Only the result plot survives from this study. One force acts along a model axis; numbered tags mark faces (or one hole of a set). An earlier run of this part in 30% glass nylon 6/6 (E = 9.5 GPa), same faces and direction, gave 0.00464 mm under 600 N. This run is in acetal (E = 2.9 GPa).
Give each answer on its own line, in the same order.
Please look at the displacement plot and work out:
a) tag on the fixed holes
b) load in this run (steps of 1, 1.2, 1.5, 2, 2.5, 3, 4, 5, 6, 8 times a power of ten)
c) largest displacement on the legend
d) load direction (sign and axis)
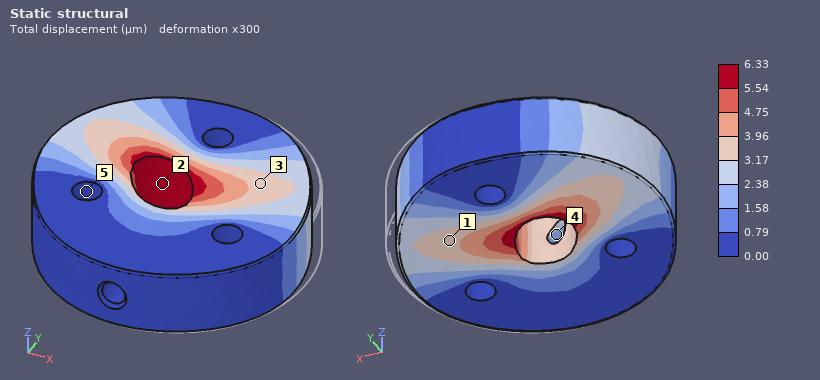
5
250 N
6.33 µm
-X
